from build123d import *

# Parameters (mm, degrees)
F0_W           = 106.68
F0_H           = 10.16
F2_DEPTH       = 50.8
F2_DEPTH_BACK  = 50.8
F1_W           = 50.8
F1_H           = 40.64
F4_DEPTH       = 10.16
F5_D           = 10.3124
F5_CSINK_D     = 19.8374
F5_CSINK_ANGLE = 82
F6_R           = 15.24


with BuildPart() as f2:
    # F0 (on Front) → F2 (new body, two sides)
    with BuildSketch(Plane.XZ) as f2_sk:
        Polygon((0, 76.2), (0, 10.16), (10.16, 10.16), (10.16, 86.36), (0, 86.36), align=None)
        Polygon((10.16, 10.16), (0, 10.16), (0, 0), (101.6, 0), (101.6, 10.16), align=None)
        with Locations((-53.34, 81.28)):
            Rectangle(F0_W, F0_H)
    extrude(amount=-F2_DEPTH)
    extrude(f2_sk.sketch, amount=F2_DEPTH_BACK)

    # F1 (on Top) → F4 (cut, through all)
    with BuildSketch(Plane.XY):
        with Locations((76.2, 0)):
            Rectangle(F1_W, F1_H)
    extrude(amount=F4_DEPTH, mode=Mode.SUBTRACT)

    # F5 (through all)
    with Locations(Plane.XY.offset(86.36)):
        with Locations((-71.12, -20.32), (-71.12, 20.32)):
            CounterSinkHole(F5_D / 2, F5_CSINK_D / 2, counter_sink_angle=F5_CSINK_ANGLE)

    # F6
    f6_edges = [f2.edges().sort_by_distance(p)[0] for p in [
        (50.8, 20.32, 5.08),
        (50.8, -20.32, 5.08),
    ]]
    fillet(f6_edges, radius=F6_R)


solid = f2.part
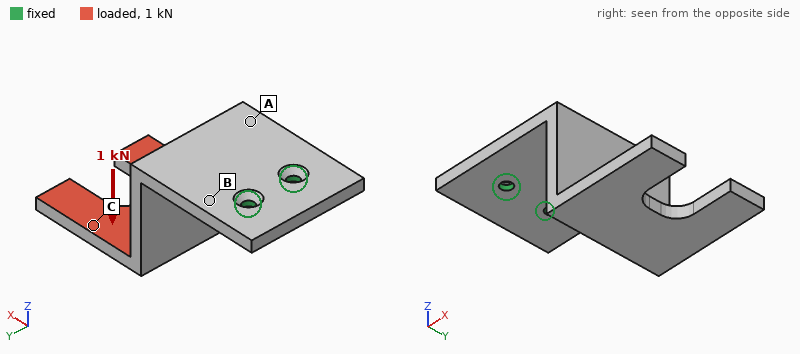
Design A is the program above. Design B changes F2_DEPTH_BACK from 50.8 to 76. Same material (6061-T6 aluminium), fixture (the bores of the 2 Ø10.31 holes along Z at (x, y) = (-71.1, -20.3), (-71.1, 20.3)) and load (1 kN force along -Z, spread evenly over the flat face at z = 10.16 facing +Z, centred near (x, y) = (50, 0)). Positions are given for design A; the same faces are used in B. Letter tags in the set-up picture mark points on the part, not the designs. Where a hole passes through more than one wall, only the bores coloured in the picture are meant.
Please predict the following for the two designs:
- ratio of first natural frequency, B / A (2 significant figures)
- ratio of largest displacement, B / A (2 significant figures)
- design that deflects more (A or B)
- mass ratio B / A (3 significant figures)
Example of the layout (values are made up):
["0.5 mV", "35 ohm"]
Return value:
["0.93", "0.90", "A", "1.27"]
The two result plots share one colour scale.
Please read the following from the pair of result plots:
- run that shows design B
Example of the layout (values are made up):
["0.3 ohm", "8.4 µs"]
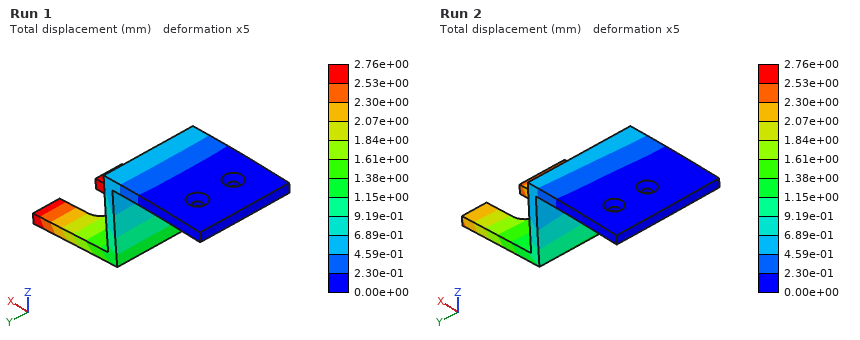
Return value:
["Run 2"]
